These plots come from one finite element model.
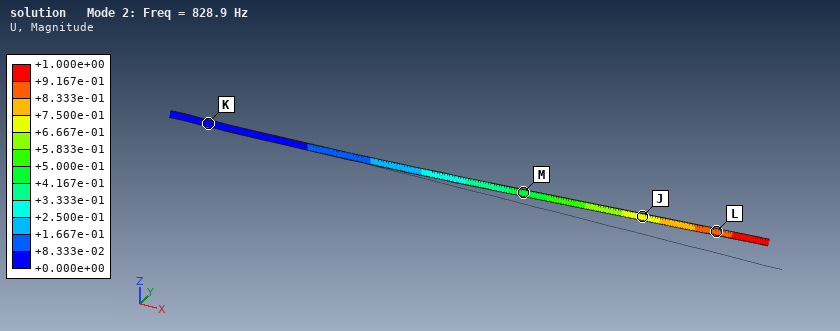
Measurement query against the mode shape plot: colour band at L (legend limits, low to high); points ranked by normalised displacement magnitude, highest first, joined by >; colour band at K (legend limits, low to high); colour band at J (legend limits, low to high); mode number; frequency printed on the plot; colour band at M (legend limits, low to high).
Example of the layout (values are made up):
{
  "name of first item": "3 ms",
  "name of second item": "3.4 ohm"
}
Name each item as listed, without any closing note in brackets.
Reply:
{
  "colour band at L": "+8.333e-01 to +9.167e-01",
  "points ranked by normalised displacement magnitude, highest first, joined by >": "L > J > M > K",
  "colour band at K": "+0.000e+00 to +8.333e-02",
  "colour band at J": "+6.667e-01 to +7.500e-01",
  "mode number": "2",
  "frequency printed on the plot": "828.9 Hz",
  "colour band at M": "+4.167e-01 to +5.000e-01"
}
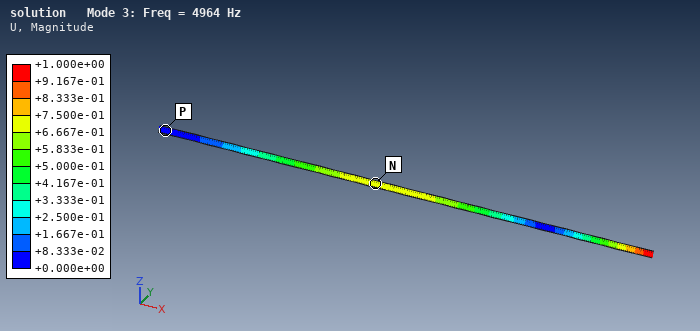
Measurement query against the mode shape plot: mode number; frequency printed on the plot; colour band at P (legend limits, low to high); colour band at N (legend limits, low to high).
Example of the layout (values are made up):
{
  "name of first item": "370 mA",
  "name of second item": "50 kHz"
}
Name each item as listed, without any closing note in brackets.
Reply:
{
  "mode number": "3",
  "frequency printed on the plot": "4964 Hz",
  "colour band at P": "+0.000e+00 to +8.333e-02",
  "colour band at N": "+6.667e-01 to +7.500e-01"
}
